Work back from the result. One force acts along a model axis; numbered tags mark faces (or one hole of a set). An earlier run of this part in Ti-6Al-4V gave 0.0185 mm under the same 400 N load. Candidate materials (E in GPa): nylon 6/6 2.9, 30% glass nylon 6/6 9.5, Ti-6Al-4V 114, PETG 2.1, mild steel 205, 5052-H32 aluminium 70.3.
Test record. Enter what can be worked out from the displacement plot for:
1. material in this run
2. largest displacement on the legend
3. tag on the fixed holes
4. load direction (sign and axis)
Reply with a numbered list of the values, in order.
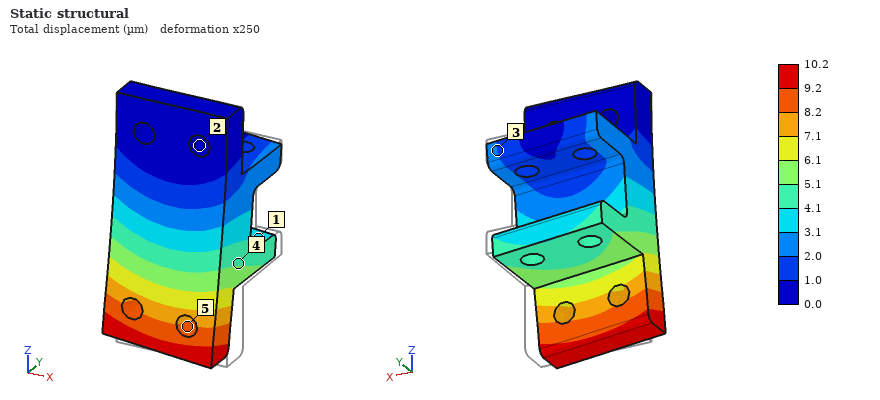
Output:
1. mild steel
2. 10.2 µm
3. 2
4. -X
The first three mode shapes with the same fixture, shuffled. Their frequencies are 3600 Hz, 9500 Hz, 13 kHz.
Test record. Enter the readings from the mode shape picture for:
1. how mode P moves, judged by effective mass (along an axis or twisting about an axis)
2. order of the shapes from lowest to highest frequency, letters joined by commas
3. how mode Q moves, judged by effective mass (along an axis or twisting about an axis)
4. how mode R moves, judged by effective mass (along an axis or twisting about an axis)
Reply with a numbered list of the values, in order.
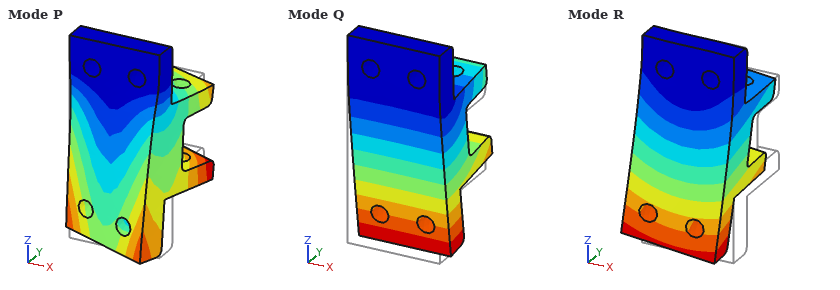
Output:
1. twisting about Z
2. Q, R, P
3. along Y
4. along X
